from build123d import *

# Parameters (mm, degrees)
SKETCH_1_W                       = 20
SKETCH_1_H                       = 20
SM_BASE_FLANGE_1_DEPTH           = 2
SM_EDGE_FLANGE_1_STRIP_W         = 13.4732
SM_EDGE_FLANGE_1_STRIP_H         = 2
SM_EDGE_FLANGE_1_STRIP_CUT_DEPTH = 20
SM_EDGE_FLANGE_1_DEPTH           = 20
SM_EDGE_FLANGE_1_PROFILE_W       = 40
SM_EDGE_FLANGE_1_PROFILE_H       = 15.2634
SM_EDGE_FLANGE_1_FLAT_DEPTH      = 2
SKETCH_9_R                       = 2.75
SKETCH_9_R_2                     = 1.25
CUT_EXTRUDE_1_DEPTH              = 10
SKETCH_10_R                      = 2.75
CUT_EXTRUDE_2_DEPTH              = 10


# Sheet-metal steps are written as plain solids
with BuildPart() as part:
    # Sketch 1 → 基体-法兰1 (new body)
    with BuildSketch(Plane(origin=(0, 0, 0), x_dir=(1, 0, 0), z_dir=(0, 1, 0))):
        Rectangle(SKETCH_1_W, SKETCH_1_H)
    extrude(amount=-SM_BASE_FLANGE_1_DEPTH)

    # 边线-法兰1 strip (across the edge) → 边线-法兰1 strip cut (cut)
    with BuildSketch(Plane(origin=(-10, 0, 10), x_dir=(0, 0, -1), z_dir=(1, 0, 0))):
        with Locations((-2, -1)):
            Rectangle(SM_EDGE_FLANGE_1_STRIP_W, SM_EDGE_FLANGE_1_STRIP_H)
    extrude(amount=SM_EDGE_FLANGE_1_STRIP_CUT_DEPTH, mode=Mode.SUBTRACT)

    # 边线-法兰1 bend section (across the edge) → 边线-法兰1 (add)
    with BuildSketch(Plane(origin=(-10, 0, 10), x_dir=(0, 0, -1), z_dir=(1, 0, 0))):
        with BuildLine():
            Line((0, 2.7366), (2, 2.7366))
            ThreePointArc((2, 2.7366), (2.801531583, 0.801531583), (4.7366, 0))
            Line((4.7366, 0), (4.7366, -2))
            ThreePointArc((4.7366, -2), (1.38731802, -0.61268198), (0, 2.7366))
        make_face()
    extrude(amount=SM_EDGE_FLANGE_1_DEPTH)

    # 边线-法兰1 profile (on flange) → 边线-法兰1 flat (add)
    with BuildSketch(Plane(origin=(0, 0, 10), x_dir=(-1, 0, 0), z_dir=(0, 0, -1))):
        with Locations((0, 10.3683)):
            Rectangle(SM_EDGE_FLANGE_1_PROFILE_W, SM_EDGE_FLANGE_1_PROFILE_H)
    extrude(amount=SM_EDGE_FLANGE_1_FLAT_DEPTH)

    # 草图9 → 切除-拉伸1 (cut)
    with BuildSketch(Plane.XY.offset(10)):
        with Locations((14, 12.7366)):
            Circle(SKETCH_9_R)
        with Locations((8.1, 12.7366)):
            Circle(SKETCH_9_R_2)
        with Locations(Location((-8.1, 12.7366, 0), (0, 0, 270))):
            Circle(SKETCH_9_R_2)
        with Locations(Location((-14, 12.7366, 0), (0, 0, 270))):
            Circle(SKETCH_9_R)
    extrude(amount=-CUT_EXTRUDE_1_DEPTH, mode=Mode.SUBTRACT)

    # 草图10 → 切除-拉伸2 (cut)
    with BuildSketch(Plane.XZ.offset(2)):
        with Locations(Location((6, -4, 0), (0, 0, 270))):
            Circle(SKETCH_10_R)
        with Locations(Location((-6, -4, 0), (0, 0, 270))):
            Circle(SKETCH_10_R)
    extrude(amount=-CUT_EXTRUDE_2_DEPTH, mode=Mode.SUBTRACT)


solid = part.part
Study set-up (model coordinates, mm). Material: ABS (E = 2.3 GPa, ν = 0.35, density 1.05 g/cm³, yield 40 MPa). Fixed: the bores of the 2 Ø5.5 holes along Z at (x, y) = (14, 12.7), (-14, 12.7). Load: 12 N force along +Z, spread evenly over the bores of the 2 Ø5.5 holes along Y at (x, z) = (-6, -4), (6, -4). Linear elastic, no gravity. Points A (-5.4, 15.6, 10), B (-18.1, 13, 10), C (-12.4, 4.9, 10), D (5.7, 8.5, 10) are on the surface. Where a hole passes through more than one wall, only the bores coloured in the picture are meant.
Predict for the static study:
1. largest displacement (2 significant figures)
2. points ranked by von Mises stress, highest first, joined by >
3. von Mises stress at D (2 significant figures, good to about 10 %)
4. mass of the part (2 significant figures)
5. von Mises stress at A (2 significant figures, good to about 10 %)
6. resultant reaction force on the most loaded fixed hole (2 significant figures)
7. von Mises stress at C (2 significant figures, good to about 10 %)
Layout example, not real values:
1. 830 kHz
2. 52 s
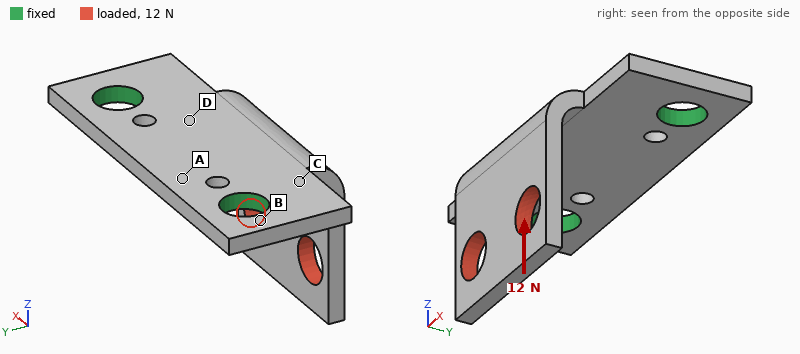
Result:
1. 0.51 mm
2. C > D > A > B
3. 3.5 MPa
4. 1.9 g
5. 1.9 MPa
6. 6.0 N
7. 5.0 MPa
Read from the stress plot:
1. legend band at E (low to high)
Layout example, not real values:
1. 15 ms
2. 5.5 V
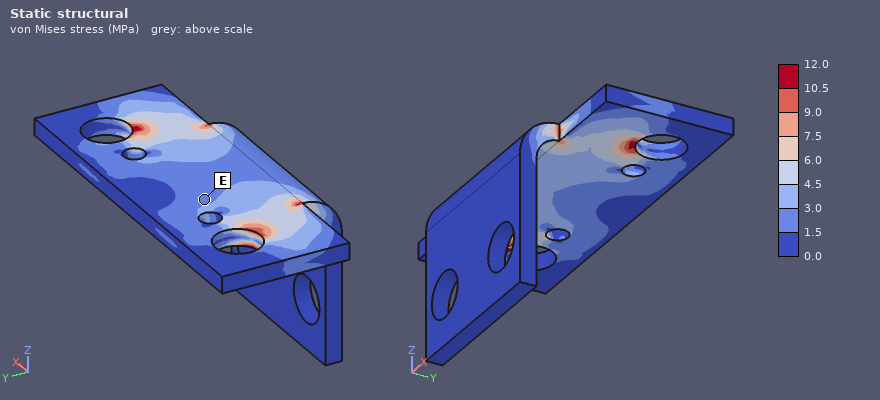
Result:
1. 1.5 to 3.0 MPa
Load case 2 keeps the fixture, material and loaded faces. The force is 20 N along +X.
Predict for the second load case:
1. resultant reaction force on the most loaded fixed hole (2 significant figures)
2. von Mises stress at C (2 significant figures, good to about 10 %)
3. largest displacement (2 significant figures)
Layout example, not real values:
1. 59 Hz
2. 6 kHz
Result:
1. 18 N
2. 4.7 MPa
3. 0.50 mm
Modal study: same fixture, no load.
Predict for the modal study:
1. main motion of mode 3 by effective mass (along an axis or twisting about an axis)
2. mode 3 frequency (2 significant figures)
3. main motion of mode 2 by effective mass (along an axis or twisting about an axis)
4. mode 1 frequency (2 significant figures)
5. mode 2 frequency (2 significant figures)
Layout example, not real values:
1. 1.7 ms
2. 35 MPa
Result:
1. along Z
2. 2000 Hz
3. along X
4. 780 Hz
5. 1600 Hz
